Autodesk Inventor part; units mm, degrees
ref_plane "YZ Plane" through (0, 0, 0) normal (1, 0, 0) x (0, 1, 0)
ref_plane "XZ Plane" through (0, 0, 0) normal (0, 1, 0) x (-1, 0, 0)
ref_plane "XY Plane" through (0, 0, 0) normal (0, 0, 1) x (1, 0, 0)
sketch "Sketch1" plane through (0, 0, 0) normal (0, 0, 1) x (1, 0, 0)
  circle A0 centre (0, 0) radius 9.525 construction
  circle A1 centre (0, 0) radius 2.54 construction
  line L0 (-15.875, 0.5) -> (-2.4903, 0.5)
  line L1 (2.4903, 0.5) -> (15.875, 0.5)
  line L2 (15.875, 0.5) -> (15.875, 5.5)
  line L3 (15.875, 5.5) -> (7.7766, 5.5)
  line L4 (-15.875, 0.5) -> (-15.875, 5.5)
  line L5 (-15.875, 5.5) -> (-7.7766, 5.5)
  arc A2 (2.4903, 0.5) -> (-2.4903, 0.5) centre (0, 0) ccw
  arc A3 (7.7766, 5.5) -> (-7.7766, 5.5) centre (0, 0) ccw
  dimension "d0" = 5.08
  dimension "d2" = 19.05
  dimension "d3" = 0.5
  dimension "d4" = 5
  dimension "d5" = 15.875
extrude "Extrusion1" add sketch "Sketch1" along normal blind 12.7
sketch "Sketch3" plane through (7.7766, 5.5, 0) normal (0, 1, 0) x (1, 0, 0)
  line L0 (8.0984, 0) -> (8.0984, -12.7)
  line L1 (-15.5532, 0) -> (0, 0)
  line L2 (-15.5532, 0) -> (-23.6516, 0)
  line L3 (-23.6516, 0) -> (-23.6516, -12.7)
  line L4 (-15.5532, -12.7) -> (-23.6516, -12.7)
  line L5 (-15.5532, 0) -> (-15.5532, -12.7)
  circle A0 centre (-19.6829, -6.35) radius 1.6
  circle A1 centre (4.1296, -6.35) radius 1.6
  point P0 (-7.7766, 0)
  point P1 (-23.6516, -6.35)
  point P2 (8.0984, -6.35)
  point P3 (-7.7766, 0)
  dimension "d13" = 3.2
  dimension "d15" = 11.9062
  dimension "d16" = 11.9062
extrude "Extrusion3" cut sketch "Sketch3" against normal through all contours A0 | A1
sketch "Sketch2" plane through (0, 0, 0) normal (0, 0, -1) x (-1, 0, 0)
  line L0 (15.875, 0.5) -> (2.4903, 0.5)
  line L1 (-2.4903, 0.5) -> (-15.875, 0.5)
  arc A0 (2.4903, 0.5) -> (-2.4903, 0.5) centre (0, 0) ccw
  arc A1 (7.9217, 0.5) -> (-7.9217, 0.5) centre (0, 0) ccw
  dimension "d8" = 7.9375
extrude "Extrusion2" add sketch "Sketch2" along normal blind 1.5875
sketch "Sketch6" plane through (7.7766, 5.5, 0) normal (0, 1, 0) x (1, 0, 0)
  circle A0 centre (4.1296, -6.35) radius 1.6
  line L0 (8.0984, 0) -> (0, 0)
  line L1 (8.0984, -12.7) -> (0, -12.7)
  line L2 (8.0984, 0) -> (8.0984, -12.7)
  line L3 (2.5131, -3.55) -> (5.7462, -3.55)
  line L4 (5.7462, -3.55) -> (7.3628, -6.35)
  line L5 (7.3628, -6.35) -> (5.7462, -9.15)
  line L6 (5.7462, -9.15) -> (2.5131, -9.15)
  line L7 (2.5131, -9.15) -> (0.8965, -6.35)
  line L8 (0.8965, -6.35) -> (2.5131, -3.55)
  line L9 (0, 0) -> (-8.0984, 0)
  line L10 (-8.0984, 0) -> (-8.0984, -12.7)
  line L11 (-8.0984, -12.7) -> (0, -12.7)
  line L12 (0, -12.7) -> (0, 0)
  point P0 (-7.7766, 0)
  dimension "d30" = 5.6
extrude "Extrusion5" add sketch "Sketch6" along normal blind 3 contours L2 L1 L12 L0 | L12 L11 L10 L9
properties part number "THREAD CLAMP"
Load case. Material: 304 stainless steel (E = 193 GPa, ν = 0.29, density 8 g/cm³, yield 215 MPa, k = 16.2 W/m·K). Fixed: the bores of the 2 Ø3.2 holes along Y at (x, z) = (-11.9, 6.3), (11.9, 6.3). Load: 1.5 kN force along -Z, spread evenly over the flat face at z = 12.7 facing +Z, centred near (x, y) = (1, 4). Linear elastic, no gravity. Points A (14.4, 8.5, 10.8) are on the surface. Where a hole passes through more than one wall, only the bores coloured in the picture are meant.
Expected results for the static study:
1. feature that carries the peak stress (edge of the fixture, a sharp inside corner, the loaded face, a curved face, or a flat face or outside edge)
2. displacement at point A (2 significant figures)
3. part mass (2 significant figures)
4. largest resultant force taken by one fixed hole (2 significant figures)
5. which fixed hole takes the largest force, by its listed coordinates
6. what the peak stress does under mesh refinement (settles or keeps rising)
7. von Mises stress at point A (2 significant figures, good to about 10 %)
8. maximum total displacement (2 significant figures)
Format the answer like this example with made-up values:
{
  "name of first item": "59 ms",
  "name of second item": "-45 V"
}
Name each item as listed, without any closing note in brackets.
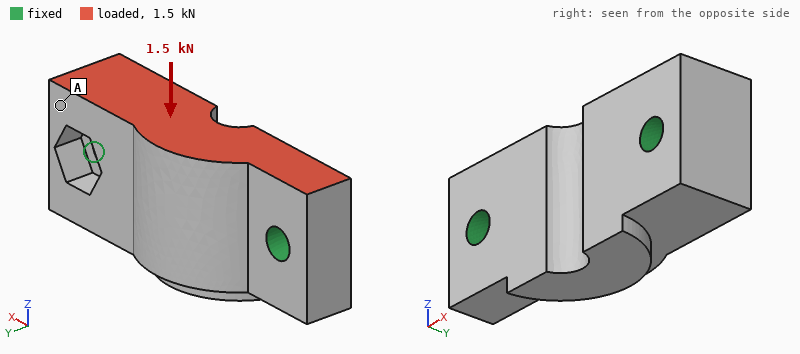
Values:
{
  "feature that carries the peak stress": "edge of the fixture",
  "displacement at point A": "0.98 µm",
  "part mass": "22 g",
  "largest resultant force taken by one fixed hole": "840 N",
  "which fixed hole takes the largest force, by its listed coordinates": "(11.9, 6.3)",
  "what the peak stress does under mesh refinement": "keeps rising",
  "von Mises stress at point A": "9.3 MPa",
  "maximum total displacement": "2.5 µm"
}
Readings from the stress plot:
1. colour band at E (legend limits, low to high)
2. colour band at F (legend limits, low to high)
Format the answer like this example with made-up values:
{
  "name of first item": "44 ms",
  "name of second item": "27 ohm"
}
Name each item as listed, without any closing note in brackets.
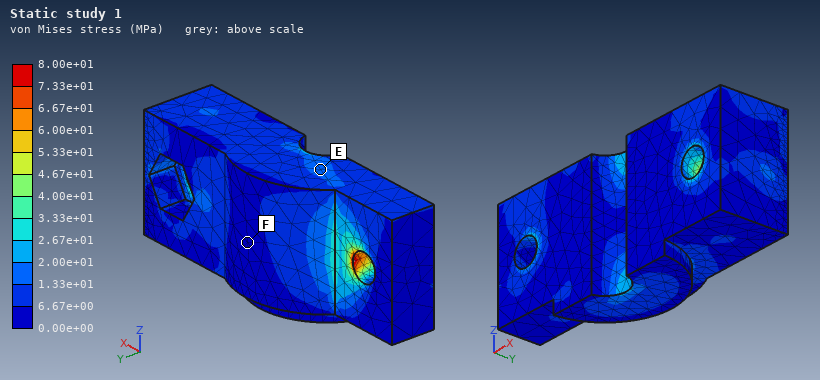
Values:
{
  "colour band at E": "1.33e+01 to 2.00e+01 MPa",
  "colour band at F": "0.00e+00 to 6.67e+00 MPa"
}
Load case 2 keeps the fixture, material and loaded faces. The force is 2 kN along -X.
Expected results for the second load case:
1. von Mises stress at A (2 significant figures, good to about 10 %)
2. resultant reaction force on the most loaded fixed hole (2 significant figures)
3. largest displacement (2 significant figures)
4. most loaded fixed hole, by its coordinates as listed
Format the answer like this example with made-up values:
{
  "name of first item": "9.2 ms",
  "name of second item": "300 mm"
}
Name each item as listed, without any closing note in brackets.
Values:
{
  "von Mises stress at A": "7.1 MPa",
  "resultant reaction force on the most loaded fixed hole": "1.2 kN",
  "largest displacement": "2.3 µm",
  "most loaded fixed hole, by its coordinates as listed": "(11.9, 6.3)"
}
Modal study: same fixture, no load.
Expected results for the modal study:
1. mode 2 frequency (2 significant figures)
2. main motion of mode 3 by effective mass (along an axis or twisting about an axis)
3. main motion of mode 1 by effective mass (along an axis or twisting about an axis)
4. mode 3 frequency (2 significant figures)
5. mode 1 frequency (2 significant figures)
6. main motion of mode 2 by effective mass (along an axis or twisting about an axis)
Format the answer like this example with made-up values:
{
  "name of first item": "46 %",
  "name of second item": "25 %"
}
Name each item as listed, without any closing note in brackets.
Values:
{
  "mode 2 frequency": "34 kHz",
  "main motion of mode 3 by effective mass": "along Z",
  "main motion of mode 1 by effective mass": "along Z",
  "mode 3 frequency": "45 kHz",
  "mode 1 frequency": "28 kHz",
  "main motion of mode 2 by effective mass": "along Y"
}
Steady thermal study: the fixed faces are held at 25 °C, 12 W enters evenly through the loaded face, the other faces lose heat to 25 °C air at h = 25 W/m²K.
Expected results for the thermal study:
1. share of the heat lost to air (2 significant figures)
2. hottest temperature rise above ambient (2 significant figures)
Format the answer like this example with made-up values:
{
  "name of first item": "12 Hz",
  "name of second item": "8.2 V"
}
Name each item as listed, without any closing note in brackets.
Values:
{
  "share of the heat lost to air": "4.4 %",
  "hottest temperature rise above ambient": "41 K"
}
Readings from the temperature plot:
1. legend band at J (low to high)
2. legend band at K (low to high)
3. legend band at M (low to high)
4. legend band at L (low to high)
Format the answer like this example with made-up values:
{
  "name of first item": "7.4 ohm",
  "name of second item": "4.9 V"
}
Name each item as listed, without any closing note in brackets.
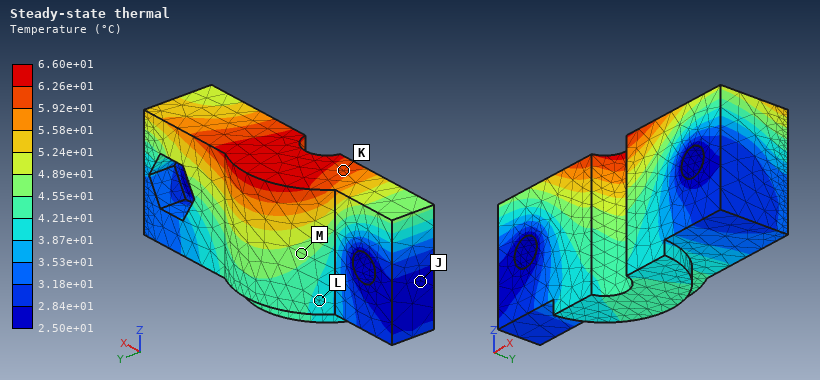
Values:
{
  "legend band at J": "2.50e+01 to 2.84e+01 °C",
  "legend band at K": "5.92e+01 to 6.26e+01 °C",
  "legend band at M": "4.55e+01 to 4.89e+01 °C",
  "legend band at L": "3.87e+01 to 4.21e+01 °C"
}
